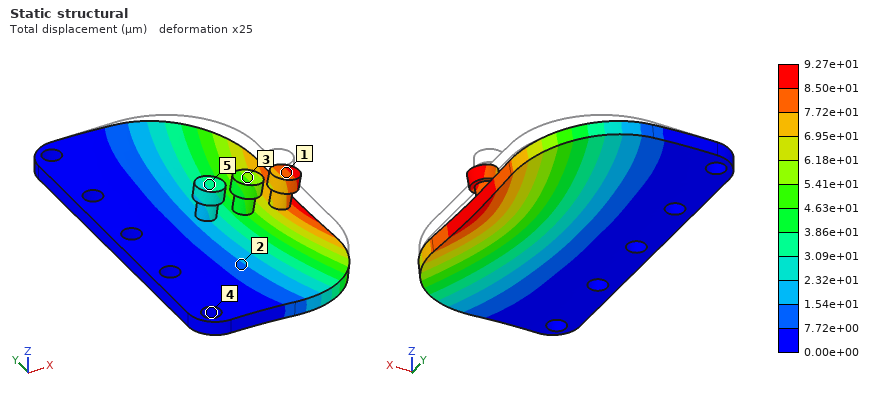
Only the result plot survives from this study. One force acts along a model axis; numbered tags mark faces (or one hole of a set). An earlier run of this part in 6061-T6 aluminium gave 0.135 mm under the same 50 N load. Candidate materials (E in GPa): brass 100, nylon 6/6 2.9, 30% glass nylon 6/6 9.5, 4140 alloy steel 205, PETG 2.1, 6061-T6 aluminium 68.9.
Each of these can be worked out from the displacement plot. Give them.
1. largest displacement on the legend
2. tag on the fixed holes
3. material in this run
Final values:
9.27e+01 µm
4
brass
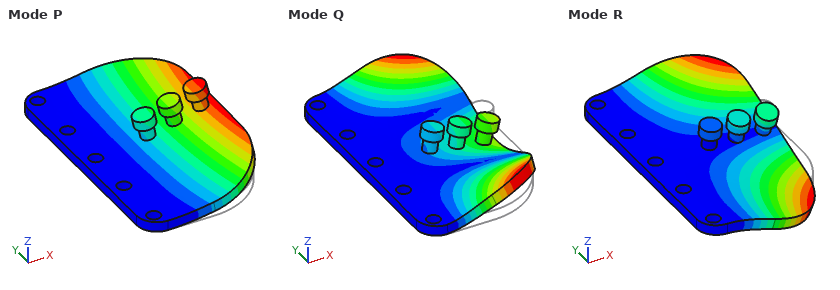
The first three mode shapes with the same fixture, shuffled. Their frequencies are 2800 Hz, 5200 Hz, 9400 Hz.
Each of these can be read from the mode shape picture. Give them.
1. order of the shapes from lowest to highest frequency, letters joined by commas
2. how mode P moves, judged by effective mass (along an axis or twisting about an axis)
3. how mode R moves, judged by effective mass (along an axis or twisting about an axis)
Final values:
P, R, Q
along Z
twisting about X
